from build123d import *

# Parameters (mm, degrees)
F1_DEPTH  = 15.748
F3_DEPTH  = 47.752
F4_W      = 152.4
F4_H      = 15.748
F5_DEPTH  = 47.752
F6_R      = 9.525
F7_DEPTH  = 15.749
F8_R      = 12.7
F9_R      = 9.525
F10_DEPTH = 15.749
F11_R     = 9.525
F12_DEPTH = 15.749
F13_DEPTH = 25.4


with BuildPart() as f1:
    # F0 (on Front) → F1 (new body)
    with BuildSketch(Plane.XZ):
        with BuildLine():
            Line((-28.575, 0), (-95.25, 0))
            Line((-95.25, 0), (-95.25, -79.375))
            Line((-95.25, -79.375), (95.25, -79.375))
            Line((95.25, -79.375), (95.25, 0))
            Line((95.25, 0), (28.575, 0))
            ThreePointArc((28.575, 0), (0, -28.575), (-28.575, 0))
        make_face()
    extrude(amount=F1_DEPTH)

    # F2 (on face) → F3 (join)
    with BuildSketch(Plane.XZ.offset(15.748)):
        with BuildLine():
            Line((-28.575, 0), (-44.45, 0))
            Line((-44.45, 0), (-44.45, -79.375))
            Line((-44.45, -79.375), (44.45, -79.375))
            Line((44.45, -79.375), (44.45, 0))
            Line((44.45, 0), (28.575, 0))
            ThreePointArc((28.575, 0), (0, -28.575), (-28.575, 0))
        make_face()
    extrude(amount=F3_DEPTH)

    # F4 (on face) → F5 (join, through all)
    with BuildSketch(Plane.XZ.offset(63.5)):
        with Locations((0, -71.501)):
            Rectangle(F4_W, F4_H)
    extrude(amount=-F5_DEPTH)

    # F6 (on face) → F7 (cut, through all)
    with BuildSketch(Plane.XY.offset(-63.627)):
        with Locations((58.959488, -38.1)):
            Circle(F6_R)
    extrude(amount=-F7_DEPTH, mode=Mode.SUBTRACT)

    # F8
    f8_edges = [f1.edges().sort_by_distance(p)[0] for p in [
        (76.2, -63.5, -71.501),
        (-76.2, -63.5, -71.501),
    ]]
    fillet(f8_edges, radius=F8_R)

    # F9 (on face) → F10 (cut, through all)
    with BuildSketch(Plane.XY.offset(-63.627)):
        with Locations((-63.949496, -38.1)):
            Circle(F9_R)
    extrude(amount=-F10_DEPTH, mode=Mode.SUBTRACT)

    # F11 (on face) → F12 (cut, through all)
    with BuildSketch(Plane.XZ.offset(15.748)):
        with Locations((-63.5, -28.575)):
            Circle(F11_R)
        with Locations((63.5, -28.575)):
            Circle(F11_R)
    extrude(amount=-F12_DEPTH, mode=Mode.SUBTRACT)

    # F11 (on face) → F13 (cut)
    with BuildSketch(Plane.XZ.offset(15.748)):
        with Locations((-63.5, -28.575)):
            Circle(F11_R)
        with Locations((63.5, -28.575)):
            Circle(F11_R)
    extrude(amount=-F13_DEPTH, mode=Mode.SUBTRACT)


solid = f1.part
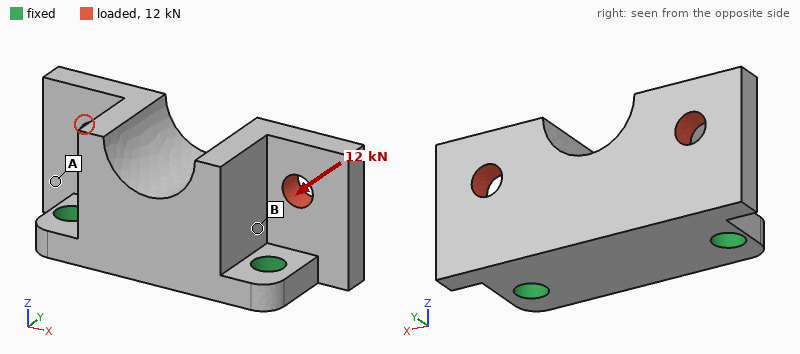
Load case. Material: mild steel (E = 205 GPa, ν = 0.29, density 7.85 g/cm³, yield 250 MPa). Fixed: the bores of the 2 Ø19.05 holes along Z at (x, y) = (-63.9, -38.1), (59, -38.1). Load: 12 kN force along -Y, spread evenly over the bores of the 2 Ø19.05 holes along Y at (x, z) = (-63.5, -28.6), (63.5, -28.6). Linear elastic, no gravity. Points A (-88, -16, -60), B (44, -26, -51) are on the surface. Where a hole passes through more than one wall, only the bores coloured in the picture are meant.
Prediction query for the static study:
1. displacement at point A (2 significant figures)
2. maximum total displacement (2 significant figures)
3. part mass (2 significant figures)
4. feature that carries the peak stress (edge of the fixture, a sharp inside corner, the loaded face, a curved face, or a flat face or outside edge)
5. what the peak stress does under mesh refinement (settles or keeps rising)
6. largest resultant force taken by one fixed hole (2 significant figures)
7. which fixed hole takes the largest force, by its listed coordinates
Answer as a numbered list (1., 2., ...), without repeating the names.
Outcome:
1. 13 µm
2. 71 µm
3. 4.1 kg
4. edge of the fixture
5. keeps rising
6. 6.3 kN
7. (59, -38.1)
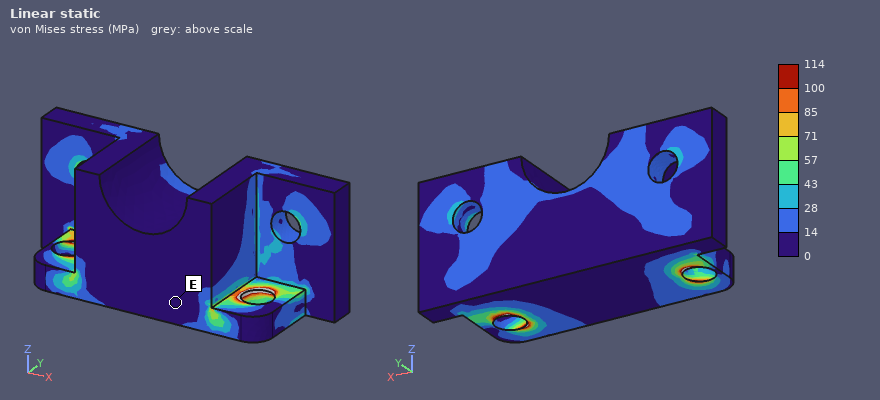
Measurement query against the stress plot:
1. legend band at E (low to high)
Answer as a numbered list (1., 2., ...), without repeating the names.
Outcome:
1. 0 to 14 MPa
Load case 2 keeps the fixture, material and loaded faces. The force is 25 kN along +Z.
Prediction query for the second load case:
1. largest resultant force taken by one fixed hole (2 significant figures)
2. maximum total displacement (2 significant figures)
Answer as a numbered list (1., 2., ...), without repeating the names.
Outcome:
1. 13 kN
2. 57 µm
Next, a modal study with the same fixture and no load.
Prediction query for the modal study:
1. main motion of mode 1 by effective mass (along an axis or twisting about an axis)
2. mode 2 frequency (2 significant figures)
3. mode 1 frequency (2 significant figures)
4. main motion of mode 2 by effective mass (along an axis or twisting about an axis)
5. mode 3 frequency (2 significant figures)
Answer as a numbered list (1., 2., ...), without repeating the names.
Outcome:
1. along Y
2. 3900 Hz
3. 1900 Hz
4. twisting about Z
5. 4700 Hz
